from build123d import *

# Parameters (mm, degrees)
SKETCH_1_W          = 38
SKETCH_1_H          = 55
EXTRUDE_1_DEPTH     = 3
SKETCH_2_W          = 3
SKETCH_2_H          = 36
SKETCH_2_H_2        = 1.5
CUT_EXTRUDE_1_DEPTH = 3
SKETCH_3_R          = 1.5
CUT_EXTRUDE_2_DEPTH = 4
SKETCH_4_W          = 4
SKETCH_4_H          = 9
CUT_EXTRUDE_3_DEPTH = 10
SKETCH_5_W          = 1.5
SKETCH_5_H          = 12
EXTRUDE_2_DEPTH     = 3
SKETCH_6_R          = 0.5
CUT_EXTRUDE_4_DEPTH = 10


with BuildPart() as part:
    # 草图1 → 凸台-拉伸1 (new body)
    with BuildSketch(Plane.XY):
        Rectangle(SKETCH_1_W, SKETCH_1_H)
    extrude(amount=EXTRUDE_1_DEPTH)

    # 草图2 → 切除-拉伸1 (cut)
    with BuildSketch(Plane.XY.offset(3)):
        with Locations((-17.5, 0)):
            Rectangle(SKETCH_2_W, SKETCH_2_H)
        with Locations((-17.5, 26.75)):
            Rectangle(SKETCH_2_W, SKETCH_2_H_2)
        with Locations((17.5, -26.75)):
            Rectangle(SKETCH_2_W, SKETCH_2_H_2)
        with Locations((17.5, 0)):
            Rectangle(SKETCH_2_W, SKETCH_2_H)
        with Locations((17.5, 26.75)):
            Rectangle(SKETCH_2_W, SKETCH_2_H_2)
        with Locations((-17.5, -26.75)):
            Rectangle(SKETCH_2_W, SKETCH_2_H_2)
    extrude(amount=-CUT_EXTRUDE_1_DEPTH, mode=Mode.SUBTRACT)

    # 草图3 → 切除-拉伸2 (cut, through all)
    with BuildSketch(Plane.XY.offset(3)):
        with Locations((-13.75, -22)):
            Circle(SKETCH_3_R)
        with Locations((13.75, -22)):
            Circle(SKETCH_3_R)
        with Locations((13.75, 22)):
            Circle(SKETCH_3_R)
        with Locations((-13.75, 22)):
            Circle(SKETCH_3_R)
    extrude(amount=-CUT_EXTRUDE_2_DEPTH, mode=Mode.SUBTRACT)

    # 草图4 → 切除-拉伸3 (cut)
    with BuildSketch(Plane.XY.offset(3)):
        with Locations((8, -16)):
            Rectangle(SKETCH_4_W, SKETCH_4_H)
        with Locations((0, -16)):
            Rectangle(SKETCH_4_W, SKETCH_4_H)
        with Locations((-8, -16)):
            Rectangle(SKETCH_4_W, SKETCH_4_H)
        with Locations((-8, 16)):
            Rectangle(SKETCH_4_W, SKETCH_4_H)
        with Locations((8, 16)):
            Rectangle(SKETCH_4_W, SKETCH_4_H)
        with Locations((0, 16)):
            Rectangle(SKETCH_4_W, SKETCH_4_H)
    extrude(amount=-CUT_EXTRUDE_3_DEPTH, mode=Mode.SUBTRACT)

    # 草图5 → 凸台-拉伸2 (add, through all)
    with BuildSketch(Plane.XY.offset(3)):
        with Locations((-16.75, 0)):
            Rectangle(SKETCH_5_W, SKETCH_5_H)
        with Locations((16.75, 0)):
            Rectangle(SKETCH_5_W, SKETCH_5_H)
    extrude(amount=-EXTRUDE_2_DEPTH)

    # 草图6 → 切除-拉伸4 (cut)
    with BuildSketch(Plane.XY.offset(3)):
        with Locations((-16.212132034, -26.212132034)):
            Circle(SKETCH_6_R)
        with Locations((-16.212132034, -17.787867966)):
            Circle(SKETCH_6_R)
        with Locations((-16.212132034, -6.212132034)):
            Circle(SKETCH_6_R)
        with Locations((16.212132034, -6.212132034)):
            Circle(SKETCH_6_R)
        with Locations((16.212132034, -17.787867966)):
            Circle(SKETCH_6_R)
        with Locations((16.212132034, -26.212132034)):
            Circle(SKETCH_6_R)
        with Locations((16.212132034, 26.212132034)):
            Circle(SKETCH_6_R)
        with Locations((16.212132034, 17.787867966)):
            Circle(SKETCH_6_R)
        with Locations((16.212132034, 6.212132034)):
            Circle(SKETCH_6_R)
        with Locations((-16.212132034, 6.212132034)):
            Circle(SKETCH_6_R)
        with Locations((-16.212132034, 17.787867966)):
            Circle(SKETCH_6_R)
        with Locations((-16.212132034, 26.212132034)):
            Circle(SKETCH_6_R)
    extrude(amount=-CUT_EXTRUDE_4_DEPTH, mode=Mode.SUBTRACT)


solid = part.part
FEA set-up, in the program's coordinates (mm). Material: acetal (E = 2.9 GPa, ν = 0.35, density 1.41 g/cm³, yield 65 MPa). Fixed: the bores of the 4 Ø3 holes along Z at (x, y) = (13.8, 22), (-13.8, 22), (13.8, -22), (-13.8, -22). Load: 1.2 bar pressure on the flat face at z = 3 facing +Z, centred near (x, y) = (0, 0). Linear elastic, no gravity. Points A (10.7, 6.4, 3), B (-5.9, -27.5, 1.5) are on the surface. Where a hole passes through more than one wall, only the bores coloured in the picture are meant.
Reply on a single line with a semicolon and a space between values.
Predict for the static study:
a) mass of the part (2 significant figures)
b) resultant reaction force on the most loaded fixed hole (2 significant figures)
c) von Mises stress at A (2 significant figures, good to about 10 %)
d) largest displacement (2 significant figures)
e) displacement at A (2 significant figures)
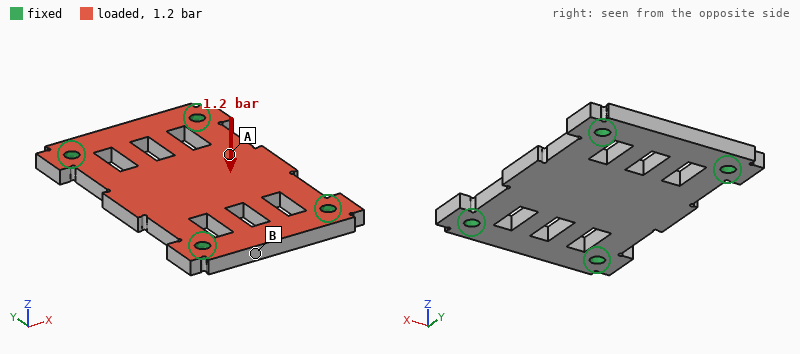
7.0 g; 49 N; 6.2 MPa; 0.25 mm; 0.21 mm
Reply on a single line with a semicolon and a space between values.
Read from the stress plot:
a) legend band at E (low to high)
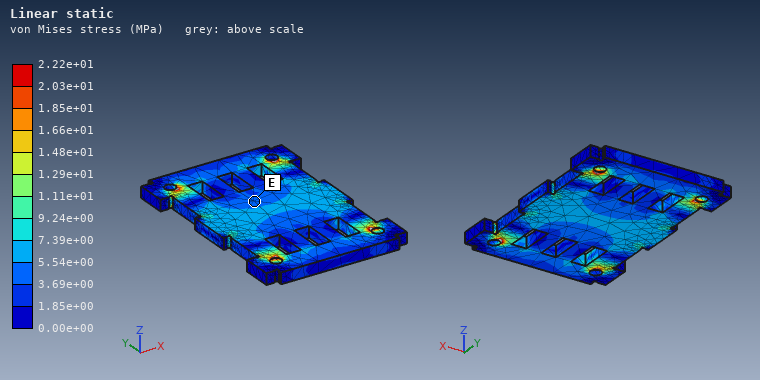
3.69e+00 to 5.54e+00 MPa
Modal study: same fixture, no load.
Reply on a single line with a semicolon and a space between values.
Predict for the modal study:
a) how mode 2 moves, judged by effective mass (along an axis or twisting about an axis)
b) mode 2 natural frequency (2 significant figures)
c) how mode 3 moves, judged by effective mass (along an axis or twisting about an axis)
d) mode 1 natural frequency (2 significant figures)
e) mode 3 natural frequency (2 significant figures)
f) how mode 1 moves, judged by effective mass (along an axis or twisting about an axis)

twisting about Y; 2600 Hz; twisting about X; 1900 Hz; 4600 Hz; along Z
